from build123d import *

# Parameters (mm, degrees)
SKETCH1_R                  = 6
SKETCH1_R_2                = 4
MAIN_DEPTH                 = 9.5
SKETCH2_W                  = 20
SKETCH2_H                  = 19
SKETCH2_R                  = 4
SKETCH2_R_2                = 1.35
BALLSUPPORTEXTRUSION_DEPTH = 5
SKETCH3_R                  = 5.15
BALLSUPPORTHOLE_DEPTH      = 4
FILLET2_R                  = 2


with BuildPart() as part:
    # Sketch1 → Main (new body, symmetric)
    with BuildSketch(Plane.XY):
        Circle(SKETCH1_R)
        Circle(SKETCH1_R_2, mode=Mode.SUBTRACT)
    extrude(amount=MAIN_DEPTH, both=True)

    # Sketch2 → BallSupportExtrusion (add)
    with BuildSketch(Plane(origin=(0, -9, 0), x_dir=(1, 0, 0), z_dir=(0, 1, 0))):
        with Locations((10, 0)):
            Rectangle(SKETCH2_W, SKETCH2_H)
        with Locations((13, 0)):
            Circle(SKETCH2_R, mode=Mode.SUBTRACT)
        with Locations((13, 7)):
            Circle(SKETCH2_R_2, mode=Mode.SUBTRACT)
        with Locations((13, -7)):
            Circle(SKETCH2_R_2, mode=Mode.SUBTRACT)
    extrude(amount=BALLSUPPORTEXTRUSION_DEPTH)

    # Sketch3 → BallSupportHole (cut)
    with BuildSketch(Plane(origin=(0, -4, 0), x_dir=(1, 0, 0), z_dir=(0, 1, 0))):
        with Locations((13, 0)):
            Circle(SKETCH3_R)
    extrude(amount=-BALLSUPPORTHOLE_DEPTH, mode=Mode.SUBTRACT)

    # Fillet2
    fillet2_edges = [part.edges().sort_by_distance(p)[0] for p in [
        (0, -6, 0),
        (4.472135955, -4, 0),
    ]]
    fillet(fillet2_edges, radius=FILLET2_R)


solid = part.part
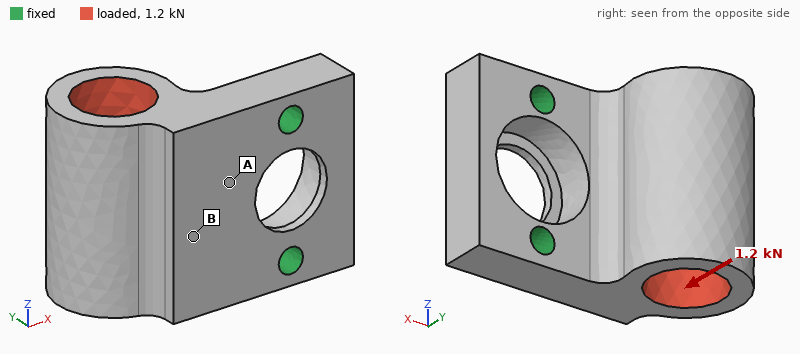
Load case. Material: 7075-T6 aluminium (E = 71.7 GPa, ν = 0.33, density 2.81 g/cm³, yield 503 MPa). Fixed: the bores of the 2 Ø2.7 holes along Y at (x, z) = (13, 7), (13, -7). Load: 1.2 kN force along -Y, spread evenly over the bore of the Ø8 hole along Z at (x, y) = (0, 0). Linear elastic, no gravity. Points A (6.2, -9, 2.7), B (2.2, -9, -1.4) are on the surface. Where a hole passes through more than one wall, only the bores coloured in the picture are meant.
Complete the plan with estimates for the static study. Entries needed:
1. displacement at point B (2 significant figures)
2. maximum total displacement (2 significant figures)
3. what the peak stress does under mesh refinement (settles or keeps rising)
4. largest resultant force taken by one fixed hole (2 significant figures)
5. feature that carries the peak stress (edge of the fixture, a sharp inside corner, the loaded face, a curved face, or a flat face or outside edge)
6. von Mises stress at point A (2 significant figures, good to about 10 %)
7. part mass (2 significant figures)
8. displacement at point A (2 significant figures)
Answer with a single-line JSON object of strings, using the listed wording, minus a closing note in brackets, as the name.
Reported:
{"displacement at point B": "0.074 mm", "maximum total displacement": "0.18 mm", "what the peak stress does under mesh refinement": "keeps rising", "largest resultant force taken by one fixed hole": "600 N", "feature that carries the peak stress": "edge of the fixture", "von Mises stress at point A": "66 MPa", "part mass": "7.3 g", "displacement at point A": "0.040 mm"}
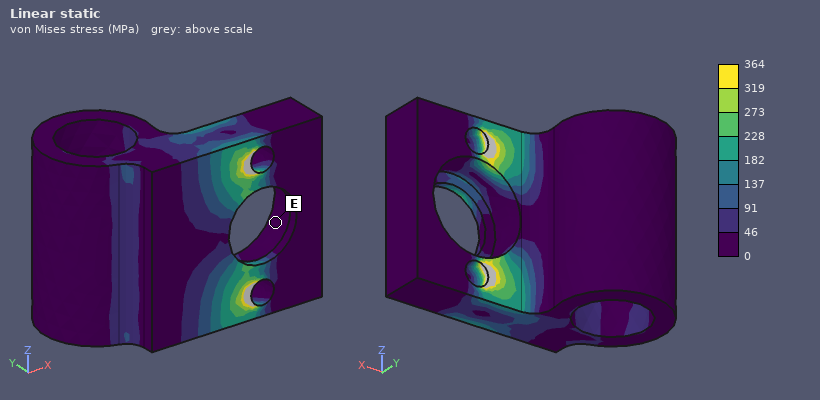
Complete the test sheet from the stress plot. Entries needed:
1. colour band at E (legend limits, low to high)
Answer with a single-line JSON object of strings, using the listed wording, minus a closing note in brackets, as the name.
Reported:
{"colour band at E": "0 to 46 MPa"}
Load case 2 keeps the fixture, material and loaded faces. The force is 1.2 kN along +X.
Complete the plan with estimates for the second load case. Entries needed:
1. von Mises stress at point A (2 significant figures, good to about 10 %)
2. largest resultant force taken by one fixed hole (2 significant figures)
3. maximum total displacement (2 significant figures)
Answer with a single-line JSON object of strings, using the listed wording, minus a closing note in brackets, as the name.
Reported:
{"von Mises stress at point A": "55 MPa", "largest resultant force taken by one fixed hole": "620 N", "maximum total displacement": "0.14 mm"}
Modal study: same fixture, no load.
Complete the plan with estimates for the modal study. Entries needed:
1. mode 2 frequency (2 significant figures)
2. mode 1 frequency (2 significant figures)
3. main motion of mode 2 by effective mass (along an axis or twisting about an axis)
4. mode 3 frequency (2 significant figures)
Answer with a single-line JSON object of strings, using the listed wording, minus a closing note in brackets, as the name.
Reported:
{"mode 2 frequency": "16 kHz", "mode 1 frequency": "6800 Hz", "main motion of mode 2 by effective mass": "along Z", "mode 3 frequency": "24 kHz"}
